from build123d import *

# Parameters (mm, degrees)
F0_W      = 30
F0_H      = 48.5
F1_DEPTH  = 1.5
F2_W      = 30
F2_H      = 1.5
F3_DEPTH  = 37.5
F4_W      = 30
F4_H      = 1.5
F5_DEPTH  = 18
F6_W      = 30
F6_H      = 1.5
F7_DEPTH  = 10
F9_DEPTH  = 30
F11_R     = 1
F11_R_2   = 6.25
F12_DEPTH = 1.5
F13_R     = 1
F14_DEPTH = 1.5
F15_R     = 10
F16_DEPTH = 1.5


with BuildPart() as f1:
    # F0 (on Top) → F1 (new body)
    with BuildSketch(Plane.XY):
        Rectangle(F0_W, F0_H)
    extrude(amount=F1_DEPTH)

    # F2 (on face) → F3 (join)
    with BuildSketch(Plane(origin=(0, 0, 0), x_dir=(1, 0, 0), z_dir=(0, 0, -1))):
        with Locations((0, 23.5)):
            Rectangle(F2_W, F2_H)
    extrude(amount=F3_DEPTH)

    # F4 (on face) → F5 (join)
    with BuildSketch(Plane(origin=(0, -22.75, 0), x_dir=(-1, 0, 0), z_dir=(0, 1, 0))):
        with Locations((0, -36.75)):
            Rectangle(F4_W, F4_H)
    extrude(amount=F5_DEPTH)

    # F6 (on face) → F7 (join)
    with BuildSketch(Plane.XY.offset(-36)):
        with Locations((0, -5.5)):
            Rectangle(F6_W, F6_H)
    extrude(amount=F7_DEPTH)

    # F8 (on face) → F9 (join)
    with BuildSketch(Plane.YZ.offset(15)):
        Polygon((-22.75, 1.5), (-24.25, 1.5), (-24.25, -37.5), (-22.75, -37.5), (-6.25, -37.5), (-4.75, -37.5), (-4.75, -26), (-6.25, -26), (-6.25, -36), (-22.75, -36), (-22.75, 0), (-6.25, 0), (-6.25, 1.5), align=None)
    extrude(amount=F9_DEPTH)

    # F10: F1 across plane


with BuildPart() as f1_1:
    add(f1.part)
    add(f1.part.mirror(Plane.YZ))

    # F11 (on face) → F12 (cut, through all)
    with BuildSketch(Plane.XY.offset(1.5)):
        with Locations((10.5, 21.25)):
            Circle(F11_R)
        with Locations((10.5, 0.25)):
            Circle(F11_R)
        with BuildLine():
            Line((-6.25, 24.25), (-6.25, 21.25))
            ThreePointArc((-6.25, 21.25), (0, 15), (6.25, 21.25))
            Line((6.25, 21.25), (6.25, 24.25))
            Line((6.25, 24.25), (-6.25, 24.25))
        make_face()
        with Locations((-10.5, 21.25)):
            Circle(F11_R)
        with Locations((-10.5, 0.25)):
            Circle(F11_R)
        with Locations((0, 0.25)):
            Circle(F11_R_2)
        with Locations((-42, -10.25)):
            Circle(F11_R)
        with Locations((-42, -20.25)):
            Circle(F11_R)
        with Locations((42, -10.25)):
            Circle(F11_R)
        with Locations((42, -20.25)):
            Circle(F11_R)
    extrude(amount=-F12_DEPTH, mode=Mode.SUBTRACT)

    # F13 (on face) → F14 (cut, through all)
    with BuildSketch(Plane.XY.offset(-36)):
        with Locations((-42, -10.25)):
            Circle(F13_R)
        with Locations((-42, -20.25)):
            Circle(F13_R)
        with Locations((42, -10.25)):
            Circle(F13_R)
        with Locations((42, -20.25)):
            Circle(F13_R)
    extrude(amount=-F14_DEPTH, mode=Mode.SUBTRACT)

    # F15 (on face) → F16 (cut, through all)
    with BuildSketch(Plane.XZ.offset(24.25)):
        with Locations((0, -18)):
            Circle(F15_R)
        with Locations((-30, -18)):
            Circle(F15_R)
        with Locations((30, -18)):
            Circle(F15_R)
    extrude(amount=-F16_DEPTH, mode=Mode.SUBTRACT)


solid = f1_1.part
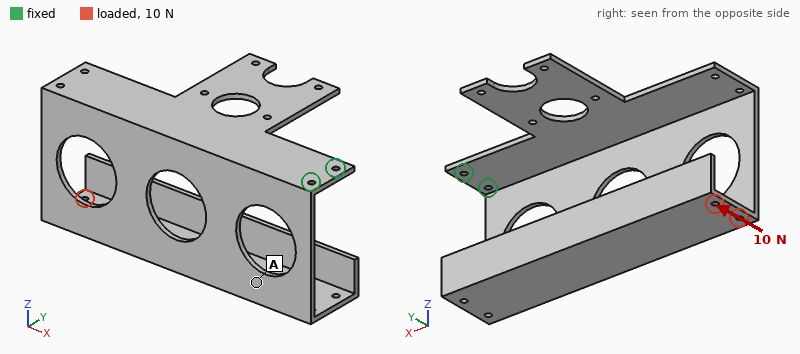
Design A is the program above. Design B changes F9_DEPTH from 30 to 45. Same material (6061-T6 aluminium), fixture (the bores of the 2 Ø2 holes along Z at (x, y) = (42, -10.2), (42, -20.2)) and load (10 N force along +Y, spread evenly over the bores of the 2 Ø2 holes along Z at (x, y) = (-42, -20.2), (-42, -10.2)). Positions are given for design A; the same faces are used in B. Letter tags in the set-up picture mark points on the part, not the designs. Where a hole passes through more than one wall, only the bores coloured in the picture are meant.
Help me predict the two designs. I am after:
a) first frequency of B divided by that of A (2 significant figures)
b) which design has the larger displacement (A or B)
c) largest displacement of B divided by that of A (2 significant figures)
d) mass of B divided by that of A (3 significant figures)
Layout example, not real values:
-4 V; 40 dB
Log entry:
1.00; A; 0.79; 1.35
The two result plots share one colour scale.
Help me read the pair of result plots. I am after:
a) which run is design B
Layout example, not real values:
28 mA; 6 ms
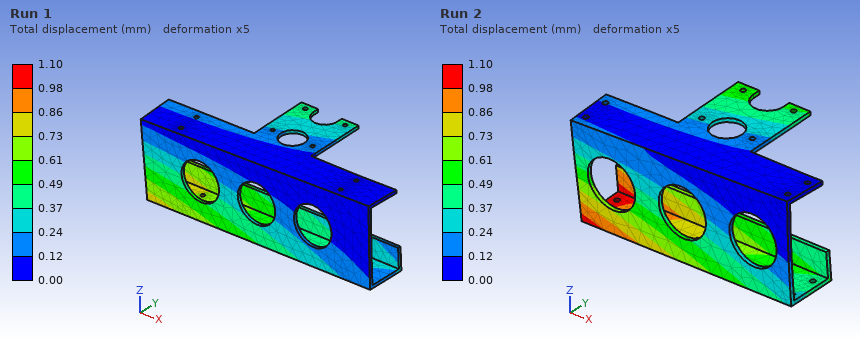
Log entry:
Run 1
